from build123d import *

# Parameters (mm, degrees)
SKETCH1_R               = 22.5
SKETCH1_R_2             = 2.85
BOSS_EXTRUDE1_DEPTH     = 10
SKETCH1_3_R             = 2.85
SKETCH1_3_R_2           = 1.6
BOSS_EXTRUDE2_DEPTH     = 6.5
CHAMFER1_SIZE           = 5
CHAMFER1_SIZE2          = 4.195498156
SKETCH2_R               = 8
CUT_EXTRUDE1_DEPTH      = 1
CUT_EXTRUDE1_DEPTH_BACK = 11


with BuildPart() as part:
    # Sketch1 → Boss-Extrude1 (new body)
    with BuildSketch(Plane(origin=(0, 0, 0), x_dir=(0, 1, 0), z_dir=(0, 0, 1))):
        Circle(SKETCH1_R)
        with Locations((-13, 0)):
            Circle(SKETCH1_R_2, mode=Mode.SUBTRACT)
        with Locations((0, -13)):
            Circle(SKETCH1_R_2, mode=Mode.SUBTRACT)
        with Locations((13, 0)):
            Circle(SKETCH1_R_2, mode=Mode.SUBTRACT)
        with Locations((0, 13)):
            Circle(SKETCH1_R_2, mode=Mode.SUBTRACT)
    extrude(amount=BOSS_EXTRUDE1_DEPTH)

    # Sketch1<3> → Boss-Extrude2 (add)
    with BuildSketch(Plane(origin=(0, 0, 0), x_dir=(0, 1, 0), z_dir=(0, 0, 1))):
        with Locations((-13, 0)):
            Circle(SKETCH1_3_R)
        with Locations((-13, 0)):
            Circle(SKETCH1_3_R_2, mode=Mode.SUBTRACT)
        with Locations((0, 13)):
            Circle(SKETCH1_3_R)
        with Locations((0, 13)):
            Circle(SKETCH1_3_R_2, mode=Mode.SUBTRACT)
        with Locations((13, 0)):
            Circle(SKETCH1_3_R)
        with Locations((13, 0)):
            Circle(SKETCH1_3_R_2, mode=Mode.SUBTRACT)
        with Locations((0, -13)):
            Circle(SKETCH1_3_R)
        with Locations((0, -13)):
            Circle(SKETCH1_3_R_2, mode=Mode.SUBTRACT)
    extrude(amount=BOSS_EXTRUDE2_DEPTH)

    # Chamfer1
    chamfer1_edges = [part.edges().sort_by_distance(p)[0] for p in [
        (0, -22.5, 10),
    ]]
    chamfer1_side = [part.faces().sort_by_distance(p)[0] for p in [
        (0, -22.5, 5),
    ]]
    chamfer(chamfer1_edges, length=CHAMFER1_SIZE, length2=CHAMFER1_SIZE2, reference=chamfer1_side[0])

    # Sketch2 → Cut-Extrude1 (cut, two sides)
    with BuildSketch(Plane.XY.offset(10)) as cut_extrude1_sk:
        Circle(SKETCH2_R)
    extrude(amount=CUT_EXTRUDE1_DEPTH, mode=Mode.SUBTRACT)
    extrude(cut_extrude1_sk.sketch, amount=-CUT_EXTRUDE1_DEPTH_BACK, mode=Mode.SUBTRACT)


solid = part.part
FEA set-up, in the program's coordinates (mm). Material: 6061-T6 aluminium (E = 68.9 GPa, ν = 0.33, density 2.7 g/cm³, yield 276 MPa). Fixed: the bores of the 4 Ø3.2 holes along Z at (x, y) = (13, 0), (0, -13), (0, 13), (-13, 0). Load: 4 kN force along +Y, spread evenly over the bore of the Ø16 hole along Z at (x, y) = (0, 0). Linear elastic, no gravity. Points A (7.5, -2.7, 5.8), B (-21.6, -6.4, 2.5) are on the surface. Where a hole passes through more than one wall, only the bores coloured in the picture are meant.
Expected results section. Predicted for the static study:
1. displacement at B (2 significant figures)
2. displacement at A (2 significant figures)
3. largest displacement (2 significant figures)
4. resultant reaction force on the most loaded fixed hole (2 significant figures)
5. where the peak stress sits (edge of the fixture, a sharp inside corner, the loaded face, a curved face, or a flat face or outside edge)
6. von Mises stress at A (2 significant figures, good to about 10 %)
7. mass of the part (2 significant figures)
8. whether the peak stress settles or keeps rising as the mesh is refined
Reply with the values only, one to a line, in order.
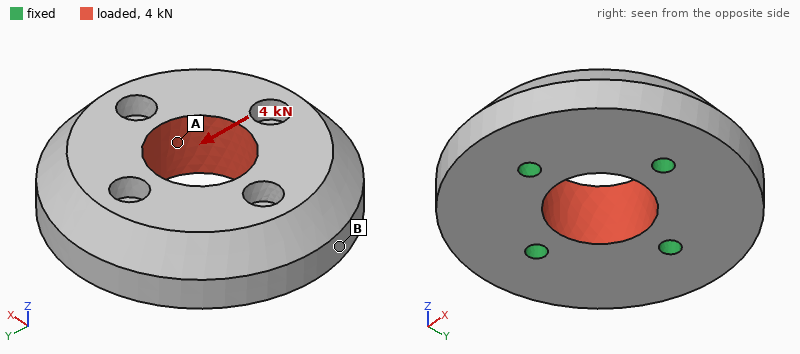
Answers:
0.58 µm
1.9 µm
3.0 µm
1.0 kN
edge of the fixture
15 MPa
32 g
keeps rising
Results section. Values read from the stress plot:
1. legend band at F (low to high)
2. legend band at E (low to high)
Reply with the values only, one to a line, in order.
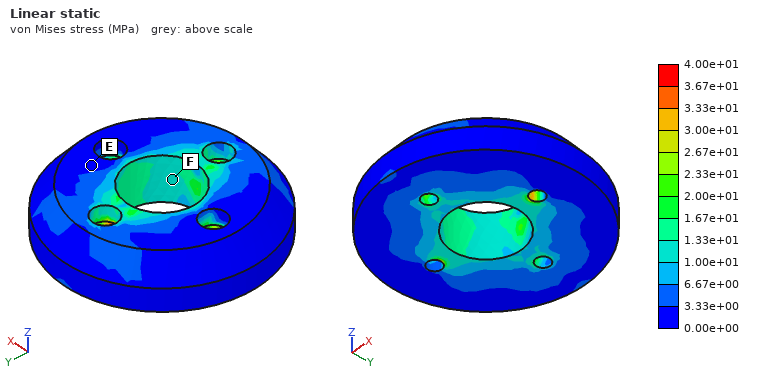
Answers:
1.00e+01 to 1.33e+01 MPa
0.00e+00 to 3.33e+00 MPa
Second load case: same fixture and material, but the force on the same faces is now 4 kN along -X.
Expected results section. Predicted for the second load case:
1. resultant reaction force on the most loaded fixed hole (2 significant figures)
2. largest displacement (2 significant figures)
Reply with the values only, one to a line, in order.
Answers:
1.0 kN
3.0 µm
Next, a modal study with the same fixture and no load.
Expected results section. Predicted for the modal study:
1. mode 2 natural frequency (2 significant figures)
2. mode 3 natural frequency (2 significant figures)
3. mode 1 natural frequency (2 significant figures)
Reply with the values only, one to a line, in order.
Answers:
29 kHz
29 kHz
27 kHz
